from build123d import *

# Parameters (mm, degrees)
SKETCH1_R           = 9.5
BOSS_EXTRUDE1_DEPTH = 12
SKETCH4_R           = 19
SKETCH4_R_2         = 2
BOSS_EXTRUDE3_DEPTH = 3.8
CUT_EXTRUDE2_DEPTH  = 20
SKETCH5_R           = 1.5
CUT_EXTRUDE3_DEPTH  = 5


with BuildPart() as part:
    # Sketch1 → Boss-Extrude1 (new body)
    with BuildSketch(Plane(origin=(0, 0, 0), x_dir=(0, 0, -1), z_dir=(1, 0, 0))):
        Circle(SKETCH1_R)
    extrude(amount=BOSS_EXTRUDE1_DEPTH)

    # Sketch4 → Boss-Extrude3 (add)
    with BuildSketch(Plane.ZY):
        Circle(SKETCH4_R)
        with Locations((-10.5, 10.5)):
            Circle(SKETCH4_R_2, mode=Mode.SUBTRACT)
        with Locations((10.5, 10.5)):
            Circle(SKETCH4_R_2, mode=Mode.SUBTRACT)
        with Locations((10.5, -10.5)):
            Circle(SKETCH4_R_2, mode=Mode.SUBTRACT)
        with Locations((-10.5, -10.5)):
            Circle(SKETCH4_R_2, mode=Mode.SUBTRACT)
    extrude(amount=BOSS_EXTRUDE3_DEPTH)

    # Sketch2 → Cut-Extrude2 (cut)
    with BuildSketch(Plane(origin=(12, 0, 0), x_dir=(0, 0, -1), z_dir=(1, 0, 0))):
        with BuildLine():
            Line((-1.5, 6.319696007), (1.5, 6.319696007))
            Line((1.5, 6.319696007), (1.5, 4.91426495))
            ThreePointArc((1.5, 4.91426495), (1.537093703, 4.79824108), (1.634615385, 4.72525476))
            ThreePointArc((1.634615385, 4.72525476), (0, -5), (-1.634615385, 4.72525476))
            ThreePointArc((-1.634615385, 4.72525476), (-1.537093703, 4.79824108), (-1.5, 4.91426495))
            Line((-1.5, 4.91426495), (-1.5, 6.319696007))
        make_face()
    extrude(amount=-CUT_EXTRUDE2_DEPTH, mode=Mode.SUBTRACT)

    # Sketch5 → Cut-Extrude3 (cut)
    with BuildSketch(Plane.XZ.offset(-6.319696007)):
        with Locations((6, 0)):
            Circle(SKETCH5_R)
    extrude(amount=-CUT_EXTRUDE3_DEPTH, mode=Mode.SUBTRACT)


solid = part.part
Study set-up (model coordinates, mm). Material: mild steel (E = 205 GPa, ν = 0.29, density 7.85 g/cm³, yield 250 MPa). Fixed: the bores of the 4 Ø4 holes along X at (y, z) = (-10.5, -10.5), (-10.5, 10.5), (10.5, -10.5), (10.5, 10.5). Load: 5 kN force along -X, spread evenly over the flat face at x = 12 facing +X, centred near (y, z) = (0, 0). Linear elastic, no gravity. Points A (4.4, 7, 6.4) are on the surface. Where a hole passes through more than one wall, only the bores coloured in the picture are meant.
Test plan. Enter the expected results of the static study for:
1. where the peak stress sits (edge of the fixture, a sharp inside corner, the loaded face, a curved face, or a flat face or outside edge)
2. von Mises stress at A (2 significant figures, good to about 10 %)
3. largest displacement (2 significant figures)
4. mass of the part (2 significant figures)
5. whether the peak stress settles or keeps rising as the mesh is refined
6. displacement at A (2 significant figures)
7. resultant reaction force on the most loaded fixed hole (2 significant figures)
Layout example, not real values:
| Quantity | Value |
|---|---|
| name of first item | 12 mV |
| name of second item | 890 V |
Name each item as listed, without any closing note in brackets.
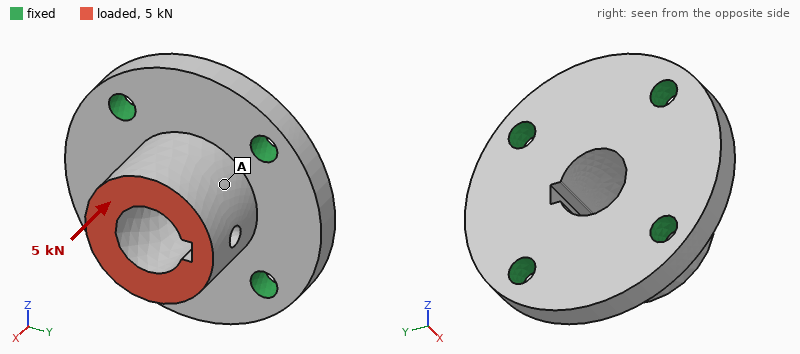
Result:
| Quantity | Value |
|---|---|
| where the peak stress sits | edge of the fixture |
| von Mises stress at A | 33 MPa |
| largest displacement | 6.8 µm |
| mass of the part | 49 g |
| whether the peak stress settles or keeps rising as the mesh is refined | keeps rising |
| displacement at A | 5.7 µm |
| resultant reaction force on the most loaded fixed hole | 1.3 kN |
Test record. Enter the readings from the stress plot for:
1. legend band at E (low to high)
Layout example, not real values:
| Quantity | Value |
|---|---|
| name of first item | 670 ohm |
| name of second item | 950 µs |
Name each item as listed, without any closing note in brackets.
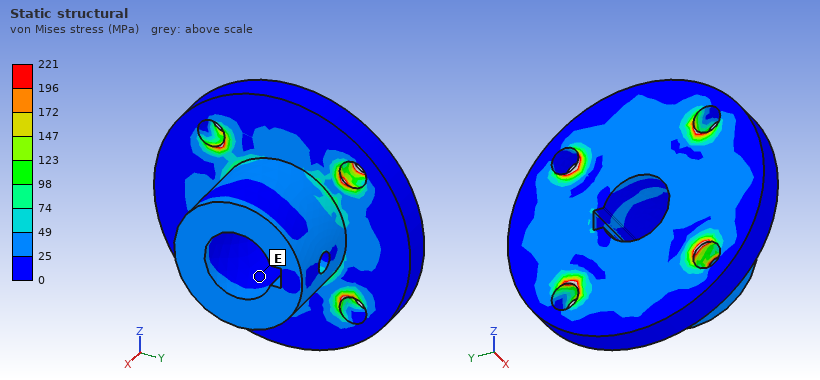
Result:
| Quantity | Value |
|---|---|
| legend band at E | 0 to 25 MPa |
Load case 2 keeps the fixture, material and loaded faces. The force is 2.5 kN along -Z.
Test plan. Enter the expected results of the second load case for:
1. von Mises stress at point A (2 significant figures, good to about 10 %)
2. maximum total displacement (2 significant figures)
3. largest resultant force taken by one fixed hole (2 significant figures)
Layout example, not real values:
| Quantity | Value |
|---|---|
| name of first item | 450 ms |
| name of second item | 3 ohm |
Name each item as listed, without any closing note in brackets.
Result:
| Quantity | Value |
|---|---|
| von Mises stress at point A | 43 MPa |
| maximum total displacement | 14 µm |
| largest resultant force taken by one fixed hole | 1.2 kN |
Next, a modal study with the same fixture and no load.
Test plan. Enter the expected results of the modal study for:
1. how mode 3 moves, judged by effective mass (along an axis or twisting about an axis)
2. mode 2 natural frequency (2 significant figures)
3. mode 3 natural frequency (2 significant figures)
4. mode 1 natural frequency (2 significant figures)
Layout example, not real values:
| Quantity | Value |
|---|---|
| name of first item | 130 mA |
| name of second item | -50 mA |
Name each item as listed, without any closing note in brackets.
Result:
| Quantity | Value |
|---|---|
| how mode 3 moves, judged by effective mass | along X |
| mode 2 natural frequency | 25 kHz |
| mode 3 natural frequency | 29 kHz |
| mode 1 natural frequency | 24 kHz |
